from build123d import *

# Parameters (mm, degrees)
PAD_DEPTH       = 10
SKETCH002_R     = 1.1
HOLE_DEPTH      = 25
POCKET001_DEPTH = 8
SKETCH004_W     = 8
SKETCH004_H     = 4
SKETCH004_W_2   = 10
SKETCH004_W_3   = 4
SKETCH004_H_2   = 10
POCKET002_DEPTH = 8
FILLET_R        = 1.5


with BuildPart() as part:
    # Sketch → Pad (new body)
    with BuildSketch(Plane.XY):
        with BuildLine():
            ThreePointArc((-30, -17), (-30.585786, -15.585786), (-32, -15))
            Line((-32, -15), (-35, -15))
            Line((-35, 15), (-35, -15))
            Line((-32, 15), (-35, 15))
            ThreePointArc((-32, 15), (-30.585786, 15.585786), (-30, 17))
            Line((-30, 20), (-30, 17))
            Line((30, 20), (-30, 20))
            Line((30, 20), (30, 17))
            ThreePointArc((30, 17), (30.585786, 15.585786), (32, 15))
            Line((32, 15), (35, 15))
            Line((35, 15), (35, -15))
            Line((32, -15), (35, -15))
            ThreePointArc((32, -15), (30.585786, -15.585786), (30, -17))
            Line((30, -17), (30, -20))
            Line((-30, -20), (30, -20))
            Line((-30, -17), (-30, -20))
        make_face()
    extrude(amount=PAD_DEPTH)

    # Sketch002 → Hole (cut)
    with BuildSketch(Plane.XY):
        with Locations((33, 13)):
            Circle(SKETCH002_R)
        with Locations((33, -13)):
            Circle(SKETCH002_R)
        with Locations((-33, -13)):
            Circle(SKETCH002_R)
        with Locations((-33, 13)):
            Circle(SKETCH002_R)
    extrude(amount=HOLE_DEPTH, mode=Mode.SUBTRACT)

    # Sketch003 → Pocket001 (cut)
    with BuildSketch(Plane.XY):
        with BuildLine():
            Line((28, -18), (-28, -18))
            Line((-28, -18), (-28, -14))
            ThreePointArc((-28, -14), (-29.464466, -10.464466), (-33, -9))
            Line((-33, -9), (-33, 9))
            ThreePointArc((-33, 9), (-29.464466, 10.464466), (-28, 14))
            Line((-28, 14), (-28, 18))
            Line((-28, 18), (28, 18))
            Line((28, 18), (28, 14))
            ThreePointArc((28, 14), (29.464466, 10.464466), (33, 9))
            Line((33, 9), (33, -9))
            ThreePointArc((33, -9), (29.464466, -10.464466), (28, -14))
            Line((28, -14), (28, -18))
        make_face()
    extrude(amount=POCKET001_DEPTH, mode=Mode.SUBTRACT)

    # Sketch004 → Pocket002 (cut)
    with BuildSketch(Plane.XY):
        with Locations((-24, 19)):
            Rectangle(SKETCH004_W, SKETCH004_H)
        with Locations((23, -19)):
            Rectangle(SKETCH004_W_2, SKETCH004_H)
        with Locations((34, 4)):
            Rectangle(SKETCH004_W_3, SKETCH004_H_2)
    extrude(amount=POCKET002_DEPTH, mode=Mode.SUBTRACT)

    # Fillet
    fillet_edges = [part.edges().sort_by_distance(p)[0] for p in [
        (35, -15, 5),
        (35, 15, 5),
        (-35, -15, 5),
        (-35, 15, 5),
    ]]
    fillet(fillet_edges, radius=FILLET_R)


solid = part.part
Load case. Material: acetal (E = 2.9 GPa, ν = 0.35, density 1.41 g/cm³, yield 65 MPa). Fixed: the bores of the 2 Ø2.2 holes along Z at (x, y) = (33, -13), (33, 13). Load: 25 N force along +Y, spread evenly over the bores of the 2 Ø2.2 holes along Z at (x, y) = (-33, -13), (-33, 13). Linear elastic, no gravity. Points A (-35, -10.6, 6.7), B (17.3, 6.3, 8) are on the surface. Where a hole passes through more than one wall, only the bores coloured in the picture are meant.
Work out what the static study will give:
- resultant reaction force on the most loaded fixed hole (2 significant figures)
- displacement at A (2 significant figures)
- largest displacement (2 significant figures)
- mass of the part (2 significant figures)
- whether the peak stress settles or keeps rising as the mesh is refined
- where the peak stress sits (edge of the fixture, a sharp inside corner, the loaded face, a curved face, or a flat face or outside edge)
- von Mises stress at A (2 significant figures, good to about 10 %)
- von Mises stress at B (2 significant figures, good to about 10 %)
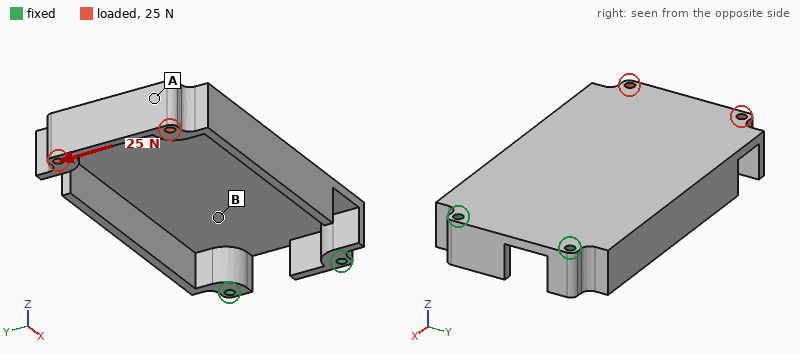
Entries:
63 N
0.61 mm
0.86 mm
12 g
keeps rising
edge of the fixture
0.92 MPa
2.5 MPa
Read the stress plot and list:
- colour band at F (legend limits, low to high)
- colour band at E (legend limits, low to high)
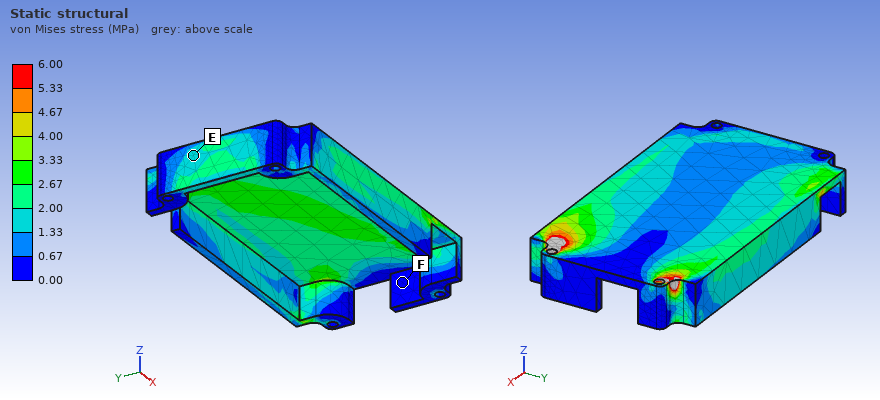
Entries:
0.00 to 0.67 MPa
1.33 to 2.00 MPa
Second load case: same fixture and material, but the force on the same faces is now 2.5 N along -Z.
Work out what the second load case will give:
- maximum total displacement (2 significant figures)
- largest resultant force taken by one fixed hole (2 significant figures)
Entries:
0.83 mm
3.5 N
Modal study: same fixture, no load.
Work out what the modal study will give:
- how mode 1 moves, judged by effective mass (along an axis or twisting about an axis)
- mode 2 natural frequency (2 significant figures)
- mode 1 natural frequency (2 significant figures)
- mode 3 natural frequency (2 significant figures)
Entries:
along Z
440 Hz
150 Hz
1200 Hz
